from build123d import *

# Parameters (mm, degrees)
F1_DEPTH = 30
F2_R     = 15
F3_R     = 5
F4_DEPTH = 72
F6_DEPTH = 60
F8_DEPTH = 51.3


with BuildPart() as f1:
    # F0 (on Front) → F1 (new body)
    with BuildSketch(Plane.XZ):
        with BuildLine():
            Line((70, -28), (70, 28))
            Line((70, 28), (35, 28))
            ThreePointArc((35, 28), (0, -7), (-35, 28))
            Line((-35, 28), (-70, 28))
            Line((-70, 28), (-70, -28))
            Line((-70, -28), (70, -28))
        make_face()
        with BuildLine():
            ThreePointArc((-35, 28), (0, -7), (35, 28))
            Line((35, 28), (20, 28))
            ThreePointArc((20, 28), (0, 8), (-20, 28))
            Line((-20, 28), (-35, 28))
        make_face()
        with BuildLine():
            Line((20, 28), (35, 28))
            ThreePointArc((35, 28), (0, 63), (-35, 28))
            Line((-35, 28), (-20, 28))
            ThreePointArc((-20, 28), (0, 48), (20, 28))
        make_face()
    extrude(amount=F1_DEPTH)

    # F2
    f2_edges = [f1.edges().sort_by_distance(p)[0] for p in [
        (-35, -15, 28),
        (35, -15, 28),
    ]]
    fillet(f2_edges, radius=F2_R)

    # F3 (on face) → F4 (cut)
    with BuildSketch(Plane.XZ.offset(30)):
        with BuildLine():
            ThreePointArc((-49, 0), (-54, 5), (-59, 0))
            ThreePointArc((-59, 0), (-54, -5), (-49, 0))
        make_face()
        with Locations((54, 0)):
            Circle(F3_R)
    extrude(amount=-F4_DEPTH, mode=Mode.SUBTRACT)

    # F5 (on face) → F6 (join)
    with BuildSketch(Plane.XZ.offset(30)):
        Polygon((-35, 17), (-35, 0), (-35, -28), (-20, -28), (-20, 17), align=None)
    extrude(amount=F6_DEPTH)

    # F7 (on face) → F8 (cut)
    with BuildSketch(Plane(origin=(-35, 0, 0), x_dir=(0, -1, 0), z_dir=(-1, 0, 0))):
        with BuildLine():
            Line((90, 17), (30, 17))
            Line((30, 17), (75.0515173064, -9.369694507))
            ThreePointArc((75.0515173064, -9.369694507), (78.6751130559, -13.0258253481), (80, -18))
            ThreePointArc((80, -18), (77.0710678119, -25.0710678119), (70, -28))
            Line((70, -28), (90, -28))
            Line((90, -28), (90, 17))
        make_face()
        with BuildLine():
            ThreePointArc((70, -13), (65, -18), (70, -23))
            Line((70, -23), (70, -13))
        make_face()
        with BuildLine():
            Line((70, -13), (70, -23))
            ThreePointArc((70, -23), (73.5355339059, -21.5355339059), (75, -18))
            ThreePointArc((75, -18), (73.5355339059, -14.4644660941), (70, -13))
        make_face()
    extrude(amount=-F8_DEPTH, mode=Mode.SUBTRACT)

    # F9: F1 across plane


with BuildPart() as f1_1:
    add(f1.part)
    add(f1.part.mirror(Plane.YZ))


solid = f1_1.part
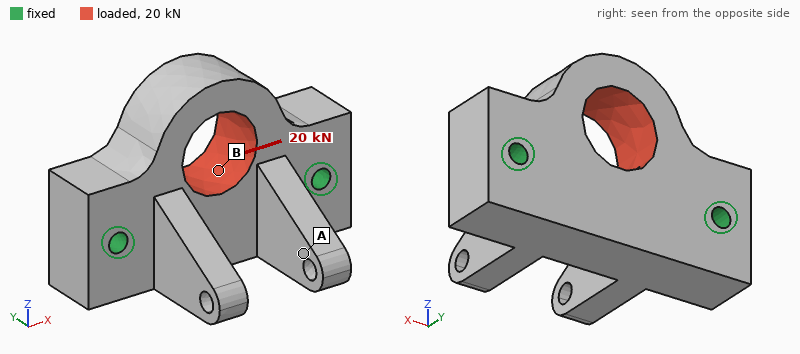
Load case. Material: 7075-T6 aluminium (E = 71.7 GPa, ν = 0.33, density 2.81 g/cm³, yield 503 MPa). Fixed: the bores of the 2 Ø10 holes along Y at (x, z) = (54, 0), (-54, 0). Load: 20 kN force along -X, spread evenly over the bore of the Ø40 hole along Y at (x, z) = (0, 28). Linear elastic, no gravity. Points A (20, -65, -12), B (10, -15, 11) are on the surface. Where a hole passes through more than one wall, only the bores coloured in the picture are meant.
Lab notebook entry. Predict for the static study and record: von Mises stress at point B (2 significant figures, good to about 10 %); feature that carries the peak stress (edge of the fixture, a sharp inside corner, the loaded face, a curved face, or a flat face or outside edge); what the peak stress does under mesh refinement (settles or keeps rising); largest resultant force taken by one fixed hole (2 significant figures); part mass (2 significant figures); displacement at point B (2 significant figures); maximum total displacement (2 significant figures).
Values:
15 MPa
edge of the fixture
keeps rising
11 kN
830 g
4.9 µm
24 µm
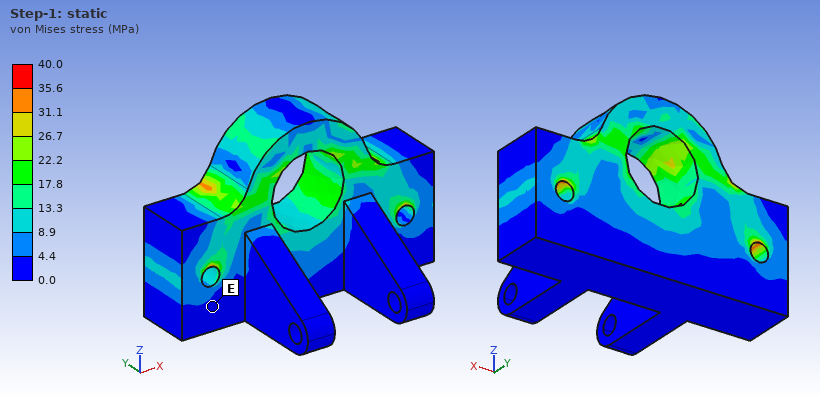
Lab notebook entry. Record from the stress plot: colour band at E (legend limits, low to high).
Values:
0.0 to 4.4 MPa
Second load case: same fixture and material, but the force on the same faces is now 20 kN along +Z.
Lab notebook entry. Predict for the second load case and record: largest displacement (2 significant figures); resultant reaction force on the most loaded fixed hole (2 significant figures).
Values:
18 µm
10 kN
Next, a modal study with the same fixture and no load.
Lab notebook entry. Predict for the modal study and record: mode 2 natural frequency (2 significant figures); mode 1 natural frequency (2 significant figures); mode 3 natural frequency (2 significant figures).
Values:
5100 Hz
4600 Hz
5600 Hz
